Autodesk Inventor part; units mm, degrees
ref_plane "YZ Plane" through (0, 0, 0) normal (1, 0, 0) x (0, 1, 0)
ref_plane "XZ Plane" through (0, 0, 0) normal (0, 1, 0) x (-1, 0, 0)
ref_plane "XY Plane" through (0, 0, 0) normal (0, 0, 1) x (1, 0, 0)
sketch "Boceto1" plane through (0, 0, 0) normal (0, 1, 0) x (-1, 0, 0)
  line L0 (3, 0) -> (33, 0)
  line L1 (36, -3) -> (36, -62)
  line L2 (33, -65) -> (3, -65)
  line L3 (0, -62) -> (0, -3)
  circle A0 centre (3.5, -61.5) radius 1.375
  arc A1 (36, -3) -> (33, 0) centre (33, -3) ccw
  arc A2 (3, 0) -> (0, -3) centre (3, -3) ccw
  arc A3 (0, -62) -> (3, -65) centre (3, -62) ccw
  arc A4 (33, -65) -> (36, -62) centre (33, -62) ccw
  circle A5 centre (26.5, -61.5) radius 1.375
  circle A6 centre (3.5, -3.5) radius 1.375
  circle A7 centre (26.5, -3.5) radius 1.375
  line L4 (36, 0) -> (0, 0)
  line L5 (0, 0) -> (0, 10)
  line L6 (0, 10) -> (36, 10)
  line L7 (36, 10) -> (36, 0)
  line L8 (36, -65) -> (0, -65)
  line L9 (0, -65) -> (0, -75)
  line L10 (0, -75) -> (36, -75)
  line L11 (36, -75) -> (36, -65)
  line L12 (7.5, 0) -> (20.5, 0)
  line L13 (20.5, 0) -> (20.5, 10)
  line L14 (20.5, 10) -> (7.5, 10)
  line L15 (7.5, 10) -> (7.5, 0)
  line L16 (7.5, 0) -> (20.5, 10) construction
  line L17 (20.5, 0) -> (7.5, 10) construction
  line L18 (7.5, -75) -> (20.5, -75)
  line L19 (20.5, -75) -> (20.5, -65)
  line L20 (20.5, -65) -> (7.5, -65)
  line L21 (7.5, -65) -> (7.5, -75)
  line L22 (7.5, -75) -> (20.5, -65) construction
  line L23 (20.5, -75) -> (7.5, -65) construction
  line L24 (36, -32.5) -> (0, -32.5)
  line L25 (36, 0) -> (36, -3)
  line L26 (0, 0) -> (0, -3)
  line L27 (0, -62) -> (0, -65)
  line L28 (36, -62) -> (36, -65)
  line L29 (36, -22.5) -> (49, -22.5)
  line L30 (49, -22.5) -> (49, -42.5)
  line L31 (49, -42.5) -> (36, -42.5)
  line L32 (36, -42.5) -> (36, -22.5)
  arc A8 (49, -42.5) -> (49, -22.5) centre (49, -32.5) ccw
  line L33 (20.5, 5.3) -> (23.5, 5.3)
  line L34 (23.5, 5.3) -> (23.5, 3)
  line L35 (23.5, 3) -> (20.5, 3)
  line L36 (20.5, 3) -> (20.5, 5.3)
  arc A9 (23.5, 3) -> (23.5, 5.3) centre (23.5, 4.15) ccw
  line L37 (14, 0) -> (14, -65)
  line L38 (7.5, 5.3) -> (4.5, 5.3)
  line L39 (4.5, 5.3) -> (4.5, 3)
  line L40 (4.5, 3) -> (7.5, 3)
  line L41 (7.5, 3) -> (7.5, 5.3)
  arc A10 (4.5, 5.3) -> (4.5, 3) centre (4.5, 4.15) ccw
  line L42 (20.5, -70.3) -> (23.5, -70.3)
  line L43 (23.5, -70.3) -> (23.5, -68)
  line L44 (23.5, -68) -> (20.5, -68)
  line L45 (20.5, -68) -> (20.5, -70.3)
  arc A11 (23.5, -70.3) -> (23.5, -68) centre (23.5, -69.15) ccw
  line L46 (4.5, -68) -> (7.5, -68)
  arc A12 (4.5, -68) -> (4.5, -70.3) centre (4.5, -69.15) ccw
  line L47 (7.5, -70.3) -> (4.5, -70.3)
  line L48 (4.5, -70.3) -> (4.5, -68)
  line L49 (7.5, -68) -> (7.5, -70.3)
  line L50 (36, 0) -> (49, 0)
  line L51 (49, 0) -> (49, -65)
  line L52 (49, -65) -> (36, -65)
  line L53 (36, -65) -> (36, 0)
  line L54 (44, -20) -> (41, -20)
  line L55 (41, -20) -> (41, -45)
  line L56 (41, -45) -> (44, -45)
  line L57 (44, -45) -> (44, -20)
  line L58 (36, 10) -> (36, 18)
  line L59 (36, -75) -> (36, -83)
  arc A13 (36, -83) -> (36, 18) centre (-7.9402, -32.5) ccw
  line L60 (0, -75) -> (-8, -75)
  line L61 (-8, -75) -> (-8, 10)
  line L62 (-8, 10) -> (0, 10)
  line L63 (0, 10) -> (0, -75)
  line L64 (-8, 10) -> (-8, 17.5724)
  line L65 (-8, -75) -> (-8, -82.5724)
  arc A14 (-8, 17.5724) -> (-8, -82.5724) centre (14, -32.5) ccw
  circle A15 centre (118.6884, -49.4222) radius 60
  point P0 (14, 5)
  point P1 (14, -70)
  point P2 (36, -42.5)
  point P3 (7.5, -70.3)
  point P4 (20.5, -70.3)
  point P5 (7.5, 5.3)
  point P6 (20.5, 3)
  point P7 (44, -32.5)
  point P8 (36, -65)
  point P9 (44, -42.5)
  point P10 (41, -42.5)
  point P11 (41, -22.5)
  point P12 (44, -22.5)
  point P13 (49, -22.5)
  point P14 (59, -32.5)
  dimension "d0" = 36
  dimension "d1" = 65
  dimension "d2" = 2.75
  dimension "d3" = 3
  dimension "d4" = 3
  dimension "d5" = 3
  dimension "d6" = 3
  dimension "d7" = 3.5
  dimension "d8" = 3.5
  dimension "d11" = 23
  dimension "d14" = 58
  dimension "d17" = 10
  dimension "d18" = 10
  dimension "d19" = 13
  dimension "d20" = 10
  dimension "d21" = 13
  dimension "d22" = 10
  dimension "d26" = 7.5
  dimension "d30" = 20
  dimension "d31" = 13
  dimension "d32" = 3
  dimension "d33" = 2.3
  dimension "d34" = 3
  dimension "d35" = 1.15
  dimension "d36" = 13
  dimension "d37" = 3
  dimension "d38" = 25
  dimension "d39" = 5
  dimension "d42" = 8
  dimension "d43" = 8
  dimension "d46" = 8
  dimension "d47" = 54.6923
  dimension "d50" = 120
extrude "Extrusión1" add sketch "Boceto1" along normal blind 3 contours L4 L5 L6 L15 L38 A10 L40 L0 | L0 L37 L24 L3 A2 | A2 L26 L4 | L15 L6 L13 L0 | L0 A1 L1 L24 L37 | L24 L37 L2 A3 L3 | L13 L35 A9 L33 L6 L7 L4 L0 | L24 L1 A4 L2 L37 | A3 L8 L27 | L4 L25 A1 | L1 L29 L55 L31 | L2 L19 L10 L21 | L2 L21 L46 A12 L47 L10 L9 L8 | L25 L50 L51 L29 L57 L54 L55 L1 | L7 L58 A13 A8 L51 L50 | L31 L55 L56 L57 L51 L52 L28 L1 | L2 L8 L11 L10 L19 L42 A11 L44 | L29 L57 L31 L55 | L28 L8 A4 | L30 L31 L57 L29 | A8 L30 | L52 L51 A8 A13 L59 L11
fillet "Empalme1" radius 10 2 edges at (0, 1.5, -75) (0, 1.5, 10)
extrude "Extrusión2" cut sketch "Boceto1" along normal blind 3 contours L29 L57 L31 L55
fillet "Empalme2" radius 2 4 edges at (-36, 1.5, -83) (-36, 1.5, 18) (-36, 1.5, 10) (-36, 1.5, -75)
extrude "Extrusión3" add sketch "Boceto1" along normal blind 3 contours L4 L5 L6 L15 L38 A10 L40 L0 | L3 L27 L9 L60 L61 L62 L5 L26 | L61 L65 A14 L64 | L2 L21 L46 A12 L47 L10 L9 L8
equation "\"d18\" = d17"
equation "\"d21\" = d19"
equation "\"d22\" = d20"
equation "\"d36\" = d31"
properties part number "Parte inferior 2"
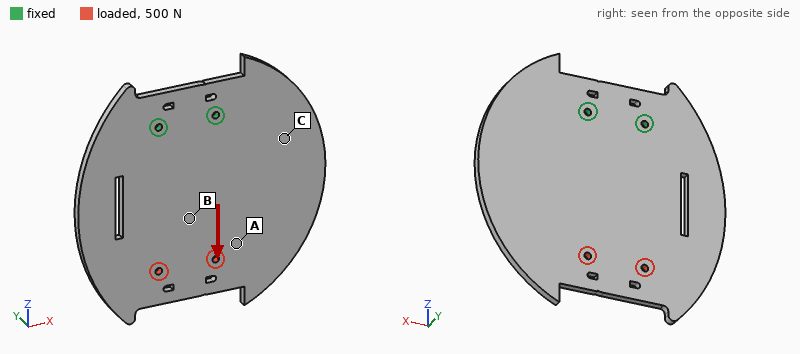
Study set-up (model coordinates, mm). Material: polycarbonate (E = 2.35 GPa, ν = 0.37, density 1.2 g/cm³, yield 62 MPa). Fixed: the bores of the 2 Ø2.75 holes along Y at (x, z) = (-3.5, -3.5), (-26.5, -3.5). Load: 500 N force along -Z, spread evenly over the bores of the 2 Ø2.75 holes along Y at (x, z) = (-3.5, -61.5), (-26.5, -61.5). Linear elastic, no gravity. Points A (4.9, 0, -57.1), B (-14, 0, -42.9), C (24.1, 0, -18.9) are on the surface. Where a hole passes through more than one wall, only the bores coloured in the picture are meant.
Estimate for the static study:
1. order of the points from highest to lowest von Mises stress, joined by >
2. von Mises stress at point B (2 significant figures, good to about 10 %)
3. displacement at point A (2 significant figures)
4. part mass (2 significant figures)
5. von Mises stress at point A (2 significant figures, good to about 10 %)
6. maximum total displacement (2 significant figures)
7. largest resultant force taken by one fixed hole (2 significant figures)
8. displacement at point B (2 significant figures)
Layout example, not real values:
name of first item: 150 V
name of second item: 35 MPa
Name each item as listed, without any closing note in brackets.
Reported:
order of the points from highest to lowest von Mises stress, joined by >: B > A > C
von Mises stress at point B: 3.6 MPa
displacement at point A: 0.078 mm
part mass: 27 g
von Mises stress at point A: 2.2 MPa
maximum total displacement: 0.11 mm
largest resultant force taken by one fixed hole: 250 N
displacement at point B: 0.069 mm
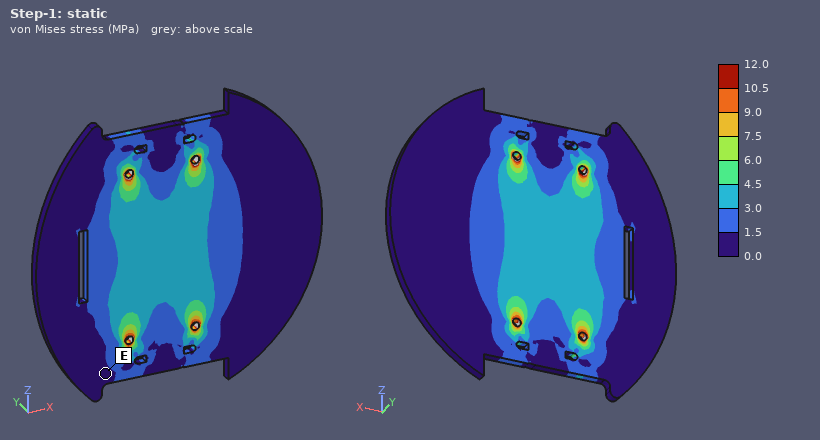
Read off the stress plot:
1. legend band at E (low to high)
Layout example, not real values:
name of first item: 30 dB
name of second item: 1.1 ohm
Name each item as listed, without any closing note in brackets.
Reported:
legend band at E: 0.0 to 1.5 MPa
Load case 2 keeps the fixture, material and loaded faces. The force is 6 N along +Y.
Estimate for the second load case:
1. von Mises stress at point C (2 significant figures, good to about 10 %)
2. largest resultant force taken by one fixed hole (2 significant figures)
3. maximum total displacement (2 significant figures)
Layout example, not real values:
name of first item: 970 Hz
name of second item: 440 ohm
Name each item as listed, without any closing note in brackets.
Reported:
von Mises stress at point C: 1.2 MPa
largest resultant force taken by one fixed hole: 3.0 N
maximum total displacement: 1.6 mm
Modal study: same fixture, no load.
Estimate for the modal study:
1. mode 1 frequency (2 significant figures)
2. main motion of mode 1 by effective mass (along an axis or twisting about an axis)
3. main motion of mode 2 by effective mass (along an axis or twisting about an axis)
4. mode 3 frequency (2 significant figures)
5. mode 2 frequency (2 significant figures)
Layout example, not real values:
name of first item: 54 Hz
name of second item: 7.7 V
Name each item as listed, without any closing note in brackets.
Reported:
mode 1 frequency: 120 Hz
main motion of mode 1 by effective mass: along Y
main motion of mode 2 by effective mass: twisting about Z
mode 3 frequency: 440 Hz
mode 2 frequency: 210 Hz
